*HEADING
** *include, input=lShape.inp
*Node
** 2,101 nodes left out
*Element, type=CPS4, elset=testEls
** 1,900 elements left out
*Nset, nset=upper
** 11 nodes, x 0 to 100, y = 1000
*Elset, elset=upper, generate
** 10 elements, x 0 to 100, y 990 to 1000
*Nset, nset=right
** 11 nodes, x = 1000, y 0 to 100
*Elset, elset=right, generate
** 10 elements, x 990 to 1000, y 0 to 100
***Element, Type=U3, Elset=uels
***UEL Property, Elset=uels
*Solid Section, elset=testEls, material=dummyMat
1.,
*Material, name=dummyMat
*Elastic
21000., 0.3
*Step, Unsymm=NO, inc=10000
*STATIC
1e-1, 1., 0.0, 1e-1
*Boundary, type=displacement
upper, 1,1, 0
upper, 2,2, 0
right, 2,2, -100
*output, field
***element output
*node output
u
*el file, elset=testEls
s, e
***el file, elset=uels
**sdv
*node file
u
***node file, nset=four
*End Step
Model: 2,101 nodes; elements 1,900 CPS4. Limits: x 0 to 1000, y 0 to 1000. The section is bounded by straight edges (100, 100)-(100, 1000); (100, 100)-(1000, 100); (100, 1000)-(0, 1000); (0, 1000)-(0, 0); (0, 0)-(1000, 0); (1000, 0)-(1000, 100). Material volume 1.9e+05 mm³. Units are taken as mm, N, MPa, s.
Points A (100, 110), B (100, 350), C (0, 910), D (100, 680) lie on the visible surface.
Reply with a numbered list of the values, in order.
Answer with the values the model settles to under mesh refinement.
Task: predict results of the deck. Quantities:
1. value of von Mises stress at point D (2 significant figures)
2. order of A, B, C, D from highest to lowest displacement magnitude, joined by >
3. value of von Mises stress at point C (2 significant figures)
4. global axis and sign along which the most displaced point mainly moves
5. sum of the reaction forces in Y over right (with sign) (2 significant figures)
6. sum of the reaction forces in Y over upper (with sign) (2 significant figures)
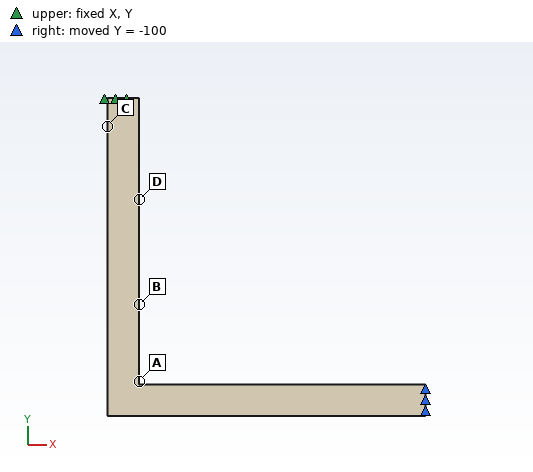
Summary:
1. 91 MPa
2. A > B > D > C
3. 87 MPa
4. -Y
5. -160 N
6. 160 N
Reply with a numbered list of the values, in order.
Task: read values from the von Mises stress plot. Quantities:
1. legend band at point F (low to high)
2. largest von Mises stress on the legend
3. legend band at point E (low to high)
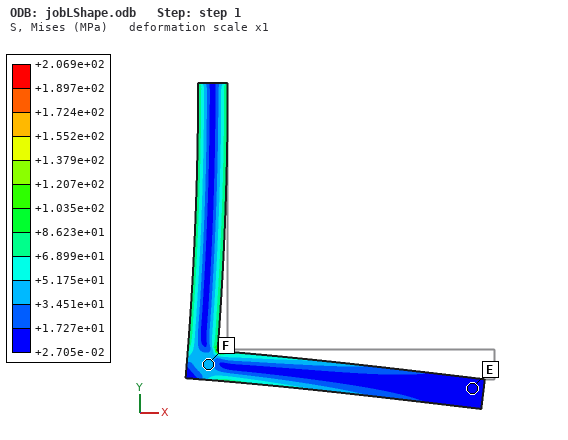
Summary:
1. +3.451e+01 to +5.175e+01 MPa
2. +2.069e+02 MPa
3. +2.705e-02 to +1.727e+01 MPa
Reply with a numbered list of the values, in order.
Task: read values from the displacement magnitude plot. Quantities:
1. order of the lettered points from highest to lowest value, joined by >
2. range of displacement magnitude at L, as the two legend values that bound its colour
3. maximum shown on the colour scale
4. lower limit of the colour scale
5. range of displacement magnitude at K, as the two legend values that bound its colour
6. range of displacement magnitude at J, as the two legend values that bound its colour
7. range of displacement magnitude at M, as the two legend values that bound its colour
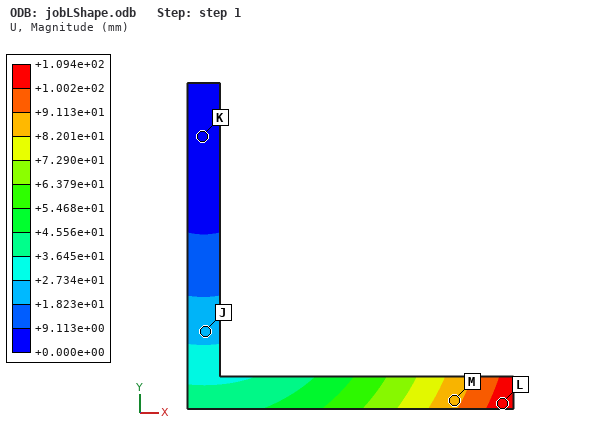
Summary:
1. L > M > J > K
2. +1.002e+02 to +1.094e+02 mm
3. +1.094e+02 mm
4. +0.000e+00 mm
5. +0.000e+00 to +9.113e+00 mm
6. +1.823e+01 to +2.734e+01 mm
7. +8.201e+01 to +9.113e+01 mm
